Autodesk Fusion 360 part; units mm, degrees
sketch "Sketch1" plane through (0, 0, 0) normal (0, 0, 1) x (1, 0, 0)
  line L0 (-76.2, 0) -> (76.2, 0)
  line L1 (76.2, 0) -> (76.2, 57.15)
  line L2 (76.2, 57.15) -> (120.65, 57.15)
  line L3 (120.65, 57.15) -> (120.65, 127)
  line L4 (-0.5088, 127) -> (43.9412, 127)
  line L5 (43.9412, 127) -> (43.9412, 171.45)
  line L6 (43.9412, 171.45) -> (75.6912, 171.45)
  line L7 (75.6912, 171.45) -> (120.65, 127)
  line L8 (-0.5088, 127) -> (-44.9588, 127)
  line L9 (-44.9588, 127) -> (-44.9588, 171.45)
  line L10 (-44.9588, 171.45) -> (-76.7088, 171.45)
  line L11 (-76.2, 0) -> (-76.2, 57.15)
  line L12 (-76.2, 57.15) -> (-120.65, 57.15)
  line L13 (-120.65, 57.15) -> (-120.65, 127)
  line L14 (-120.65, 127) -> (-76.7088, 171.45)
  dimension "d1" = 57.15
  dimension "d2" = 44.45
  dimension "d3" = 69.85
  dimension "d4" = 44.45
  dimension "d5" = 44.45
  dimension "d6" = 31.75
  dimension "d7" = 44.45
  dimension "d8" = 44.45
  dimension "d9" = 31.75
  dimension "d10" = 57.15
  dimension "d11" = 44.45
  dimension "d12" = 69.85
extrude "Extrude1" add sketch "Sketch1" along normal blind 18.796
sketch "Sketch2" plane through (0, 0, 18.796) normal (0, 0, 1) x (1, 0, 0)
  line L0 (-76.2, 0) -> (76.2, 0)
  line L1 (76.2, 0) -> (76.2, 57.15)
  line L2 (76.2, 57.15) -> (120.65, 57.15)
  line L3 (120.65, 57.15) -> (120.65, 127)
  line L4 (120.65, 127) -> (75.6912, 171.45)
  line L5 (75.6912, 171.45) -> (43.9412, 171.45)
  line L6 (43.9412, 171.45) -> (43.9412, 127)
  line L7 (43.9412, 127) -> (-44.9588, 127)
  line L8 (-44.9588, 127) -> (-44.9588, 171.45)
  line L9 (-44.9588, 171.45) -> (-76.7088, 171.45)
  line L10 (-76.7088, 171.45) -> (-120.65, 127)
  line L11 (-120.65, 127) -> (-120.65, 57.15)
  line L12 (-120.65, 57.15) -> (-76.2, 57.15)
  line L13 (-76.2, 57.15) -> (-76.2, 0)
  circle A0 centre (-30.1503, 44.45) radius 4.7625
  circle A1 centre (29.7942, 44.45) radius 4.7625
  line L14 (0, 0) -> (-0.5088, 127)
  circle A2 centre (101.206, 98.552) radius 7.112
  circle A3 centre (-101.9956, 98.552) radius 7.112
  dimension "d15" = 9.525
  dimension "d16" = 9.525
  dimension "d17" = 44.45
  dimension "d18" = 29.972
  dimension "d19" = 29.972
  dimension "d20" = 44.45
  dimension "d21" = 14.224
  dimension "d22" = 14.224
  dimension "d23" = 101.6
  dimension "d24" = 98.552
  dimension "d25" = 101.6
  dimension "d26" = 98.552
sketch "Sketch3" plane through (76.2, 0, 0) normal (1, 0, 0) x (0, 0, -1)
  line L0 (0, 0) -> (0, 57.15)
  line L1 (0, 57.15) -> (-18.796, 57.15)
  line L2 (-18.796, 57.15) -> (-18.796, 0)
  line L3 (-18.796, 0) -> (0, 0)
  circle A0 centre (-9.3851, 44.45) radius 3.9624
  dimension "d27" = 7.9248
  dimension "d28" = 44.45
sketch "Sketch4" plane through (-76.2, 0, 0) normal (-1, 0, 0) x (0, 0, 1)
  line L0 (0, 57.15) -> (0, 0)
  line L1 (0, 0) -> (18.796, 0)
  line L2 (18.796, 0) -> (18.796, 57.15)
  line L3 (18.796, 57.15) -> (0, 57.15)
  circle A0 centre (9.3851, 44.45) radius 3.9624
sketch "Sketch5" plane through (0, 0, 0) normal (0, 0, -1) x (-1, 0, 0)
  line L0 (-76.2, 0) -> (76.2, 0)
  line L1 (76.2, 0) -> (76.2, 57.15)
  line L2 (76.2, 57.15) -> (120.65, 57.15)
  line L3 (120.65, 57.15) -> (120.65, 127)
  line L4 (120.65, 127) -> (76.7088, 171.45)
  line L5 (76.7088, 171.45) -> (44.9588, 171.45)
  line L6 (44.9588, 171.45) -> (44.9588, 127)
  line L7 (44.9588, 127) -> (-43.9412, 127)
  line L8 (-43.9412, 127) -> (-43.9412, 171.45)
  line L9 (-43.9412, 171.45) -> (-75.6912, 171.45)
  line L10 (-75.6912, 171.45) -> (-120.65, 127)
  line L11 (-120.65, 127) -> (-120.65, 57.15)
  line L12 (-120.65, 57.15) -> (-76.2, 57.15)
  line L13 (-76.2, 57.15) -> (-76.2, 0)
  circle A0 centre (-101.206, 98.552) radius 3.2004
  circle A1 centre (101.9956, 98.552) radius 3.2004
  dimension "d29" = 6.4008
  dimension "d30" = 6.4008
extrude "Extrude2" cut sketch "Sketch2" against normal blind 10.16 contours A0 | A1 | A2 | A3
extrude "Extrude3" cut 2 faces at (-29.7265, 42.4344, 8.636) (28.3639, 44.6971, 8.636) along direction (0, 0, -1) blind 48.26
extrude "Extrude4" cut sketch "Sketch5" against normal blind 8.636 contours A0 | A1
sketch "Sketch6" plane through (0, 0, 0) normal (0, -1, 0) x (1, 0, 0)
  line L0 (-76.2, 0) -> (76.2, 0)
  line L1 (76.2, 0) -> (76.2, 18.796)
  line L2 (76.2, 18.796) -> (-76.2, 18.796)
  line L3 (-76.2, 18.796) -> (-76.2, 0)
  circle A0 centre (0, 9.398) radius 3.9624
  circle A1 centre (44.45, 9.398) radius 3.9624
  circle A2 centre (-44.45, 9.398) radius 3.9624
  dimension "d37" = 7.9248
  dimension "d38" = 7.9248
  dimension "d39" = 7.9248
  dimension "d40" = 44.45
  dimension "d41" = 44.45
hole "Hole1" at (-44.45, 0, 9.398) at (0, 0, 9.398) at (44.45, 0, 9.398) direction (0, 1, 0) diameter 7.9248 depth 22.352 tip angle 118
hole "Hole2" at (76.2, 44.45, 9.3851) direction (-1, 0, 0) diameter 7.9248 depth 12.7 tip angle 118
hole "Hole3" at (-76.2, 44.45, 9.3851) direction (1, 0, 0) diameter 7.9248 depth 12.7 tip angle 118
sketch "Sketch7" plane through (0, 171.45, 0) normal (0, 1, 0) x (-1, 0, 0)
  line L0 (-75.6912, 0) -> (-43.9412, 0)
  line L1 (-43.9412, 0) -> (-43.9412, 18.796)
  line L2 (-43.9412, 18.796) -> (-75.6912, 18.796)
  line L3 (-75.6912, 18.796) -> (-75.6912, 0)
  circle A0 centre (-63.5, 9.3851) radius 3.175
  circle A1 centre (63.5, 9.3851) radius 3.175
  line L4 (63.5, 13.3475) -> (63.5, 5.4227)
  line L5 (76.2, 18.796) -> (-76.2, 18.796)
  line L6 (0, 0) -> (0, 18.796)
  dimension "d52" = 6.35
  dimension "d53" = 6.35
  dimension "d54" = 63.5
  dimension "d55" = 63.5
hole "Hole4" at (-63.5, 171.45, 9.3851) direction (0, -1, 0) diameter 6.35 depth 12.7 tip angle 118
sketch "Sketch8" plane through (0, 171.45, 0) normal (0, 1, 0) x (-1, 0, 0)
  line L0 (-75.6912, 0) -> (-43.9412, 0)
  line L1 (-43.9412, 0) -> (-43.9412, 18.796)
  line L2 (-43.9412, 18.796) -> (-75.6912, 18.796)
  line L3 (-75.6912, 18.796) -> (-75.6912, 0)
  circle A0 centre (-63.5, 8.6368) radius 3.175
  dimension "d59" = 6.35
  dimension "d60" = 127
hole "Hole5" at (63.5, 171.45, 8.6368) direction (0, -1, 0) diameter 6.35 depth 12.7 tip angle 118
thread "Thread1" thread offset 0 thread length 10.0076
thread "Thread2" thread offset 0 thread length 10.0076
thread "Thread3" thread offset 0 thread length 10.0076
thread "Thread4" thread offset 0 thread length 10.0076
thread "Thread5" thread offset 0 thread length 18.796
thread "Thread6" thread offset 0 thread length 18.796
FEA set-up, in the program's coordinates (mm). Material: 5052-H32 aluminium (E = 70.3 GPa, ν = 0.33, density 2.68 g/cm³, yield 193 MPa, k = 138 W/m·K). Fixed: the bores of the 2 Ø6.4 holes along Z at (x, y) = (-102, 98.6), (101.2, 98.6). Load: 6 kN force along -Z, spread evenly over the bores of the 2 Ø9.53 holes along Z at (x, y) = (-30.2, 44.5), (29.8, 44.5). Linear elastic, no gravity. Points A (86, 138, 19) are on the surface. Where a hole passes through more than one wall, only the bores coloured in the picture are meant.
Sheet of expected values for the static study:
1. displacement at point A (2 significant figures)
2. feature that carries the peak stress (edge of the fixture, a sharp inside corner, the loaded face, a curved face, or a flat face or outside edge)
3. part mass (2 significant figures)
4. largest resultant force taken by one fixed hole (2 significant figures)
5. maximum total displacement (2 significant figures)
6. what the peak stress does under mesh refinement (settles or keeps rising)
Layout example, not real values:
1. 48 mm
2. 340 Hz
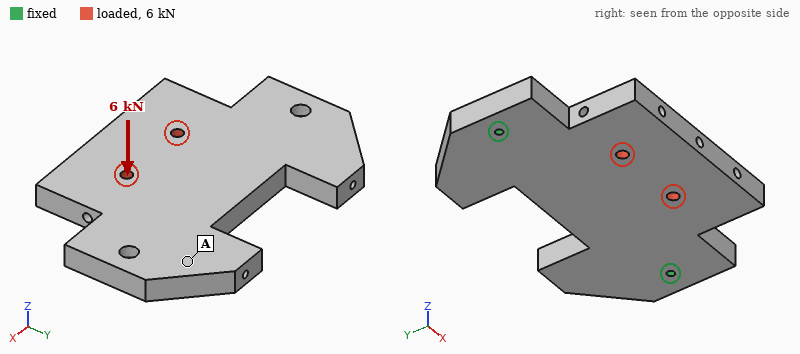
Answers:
1. 0.22 mm
2. edge of the fixture
3. 1.5 kg
4. 5.4 kN
5. 0.91 mm
6. keeps rising
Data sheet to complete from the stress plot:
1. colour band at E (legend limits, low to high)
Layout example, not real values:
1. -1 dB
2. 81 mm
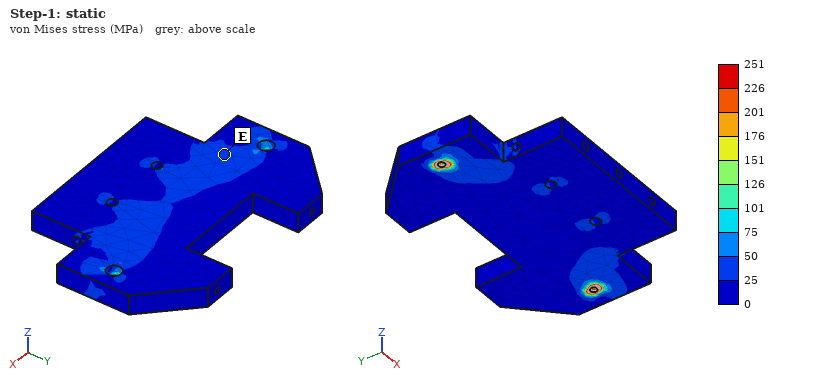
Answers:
1. 25 to 50 MPa
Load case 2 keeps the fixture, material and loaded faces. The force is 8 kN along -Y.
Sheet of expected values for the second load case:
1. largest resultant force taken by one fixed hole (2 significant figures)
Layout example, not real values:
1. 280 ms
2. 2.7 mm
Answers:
1. 4.3 kN
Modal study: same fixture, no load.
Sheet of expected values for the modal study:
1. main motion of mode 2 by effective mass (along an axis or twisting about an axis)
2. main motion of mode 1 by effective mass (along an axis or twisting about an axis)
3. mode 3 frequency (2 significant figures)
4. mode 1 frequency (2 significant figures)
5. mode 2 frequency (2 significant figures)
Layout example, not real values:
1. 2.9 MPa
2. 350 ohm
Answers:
1. along Z
2. along Z
3. 1900 Hz
4. 580 Hz
5. 1300 Hz
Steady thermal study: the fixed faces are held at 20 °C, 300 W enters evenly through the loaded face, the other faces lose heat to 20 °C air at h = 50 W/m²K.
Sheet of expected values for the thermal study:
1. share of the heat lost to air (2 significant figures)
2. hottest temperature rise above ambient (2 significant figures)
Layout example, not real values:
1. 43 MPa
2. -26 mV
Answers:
1. 47 %
2. 71 K
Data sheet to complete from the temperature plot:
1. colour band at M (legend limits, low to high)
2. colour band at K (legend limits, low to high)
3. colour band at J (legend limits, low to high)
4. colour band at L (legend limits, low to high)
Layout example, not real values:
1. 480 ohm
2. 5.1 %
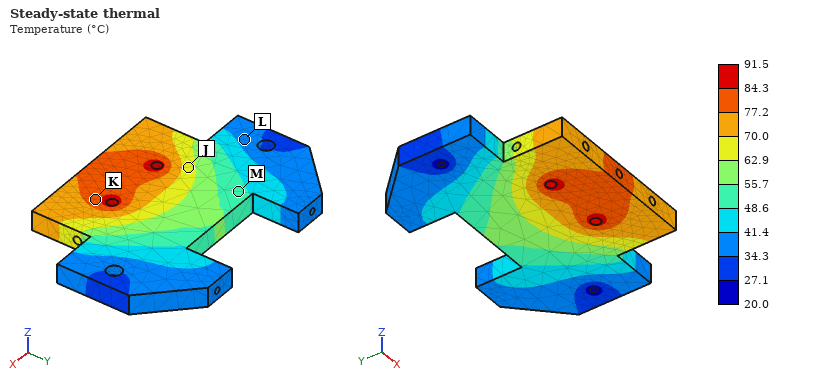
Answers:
1. 48.6 to 55.7 °C
2. 77.2 to 84.3 °C
3. 62.9 to 70.0 °C
4. 34.3 to 41.4 °C
